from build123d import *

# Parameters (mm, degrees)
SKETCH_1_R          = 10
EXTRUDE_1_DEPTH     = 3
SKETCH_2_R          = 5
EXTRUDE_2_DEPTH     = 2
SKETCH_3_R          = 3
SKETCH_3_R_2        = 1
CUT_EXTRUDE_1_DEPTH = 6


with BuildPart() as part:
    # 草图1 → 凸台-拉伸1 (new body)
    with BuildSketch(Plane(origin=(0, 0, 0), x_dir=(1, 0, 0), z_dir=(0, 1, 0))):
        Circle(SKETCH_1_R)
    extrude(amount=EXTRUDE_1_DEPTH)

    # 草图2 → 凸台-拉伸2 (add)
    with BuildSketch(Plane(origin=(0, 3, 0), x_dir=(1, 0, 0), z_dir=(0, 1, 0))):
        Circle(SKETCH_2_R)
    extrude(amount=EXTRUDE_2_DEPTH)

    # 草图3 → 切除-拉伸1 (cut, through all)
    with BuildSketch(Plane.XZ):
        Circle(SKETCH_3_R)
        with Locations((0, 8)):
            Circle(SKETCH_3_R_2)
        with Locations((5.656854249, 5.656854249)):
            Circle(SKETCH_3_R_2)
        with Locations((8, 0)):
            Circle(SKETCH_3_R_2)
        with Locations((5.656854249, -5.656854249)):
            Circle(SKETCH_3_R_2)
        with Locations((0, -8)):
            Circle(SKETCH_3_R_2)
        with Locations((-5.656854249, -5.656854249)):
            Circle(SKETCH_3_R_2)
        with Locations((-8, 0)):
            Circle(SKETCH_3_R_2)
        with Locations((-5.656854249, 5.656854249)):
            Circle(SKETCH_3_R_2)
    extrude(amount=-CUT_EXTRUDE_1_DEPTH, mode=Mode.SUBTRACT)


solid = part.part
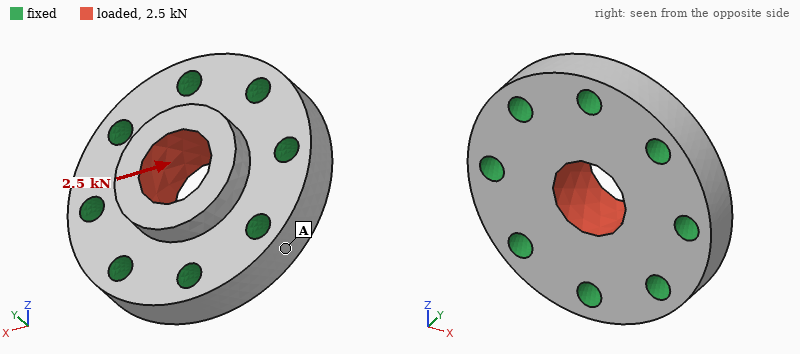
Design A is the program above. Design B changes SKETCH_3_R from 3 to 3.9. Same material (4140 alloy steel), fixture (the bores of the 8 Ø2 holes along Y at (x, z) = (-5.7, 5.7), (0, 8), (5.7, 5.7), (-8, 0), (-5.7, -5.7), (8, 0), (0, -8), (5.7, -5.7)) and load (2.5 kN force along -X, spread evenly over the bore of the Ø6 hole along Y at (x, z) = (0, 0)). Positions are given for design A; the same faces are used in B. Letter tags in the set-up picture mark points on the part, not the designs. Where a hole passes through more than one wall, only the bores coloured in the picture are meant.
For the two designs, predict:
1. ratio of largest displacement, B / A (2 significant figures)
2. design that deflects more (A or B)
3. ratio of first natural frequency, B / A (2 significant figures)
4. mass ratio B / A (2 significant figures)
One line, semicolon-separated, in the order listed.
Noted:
1.6; B; 1.2; 0.89
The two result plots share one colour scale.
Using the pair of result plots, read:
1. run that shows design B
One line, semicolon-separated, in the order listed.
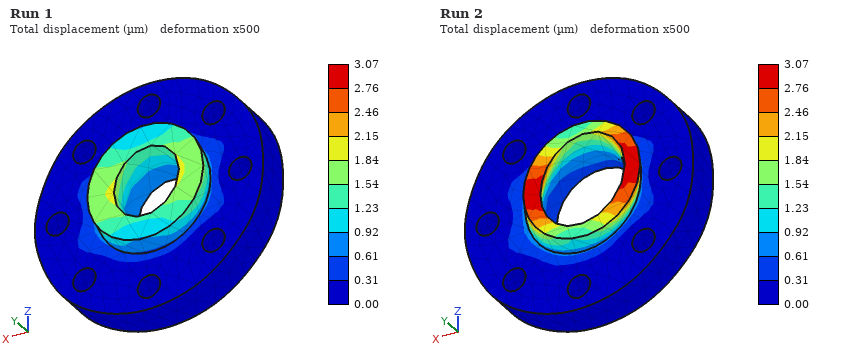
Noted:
Run 2
